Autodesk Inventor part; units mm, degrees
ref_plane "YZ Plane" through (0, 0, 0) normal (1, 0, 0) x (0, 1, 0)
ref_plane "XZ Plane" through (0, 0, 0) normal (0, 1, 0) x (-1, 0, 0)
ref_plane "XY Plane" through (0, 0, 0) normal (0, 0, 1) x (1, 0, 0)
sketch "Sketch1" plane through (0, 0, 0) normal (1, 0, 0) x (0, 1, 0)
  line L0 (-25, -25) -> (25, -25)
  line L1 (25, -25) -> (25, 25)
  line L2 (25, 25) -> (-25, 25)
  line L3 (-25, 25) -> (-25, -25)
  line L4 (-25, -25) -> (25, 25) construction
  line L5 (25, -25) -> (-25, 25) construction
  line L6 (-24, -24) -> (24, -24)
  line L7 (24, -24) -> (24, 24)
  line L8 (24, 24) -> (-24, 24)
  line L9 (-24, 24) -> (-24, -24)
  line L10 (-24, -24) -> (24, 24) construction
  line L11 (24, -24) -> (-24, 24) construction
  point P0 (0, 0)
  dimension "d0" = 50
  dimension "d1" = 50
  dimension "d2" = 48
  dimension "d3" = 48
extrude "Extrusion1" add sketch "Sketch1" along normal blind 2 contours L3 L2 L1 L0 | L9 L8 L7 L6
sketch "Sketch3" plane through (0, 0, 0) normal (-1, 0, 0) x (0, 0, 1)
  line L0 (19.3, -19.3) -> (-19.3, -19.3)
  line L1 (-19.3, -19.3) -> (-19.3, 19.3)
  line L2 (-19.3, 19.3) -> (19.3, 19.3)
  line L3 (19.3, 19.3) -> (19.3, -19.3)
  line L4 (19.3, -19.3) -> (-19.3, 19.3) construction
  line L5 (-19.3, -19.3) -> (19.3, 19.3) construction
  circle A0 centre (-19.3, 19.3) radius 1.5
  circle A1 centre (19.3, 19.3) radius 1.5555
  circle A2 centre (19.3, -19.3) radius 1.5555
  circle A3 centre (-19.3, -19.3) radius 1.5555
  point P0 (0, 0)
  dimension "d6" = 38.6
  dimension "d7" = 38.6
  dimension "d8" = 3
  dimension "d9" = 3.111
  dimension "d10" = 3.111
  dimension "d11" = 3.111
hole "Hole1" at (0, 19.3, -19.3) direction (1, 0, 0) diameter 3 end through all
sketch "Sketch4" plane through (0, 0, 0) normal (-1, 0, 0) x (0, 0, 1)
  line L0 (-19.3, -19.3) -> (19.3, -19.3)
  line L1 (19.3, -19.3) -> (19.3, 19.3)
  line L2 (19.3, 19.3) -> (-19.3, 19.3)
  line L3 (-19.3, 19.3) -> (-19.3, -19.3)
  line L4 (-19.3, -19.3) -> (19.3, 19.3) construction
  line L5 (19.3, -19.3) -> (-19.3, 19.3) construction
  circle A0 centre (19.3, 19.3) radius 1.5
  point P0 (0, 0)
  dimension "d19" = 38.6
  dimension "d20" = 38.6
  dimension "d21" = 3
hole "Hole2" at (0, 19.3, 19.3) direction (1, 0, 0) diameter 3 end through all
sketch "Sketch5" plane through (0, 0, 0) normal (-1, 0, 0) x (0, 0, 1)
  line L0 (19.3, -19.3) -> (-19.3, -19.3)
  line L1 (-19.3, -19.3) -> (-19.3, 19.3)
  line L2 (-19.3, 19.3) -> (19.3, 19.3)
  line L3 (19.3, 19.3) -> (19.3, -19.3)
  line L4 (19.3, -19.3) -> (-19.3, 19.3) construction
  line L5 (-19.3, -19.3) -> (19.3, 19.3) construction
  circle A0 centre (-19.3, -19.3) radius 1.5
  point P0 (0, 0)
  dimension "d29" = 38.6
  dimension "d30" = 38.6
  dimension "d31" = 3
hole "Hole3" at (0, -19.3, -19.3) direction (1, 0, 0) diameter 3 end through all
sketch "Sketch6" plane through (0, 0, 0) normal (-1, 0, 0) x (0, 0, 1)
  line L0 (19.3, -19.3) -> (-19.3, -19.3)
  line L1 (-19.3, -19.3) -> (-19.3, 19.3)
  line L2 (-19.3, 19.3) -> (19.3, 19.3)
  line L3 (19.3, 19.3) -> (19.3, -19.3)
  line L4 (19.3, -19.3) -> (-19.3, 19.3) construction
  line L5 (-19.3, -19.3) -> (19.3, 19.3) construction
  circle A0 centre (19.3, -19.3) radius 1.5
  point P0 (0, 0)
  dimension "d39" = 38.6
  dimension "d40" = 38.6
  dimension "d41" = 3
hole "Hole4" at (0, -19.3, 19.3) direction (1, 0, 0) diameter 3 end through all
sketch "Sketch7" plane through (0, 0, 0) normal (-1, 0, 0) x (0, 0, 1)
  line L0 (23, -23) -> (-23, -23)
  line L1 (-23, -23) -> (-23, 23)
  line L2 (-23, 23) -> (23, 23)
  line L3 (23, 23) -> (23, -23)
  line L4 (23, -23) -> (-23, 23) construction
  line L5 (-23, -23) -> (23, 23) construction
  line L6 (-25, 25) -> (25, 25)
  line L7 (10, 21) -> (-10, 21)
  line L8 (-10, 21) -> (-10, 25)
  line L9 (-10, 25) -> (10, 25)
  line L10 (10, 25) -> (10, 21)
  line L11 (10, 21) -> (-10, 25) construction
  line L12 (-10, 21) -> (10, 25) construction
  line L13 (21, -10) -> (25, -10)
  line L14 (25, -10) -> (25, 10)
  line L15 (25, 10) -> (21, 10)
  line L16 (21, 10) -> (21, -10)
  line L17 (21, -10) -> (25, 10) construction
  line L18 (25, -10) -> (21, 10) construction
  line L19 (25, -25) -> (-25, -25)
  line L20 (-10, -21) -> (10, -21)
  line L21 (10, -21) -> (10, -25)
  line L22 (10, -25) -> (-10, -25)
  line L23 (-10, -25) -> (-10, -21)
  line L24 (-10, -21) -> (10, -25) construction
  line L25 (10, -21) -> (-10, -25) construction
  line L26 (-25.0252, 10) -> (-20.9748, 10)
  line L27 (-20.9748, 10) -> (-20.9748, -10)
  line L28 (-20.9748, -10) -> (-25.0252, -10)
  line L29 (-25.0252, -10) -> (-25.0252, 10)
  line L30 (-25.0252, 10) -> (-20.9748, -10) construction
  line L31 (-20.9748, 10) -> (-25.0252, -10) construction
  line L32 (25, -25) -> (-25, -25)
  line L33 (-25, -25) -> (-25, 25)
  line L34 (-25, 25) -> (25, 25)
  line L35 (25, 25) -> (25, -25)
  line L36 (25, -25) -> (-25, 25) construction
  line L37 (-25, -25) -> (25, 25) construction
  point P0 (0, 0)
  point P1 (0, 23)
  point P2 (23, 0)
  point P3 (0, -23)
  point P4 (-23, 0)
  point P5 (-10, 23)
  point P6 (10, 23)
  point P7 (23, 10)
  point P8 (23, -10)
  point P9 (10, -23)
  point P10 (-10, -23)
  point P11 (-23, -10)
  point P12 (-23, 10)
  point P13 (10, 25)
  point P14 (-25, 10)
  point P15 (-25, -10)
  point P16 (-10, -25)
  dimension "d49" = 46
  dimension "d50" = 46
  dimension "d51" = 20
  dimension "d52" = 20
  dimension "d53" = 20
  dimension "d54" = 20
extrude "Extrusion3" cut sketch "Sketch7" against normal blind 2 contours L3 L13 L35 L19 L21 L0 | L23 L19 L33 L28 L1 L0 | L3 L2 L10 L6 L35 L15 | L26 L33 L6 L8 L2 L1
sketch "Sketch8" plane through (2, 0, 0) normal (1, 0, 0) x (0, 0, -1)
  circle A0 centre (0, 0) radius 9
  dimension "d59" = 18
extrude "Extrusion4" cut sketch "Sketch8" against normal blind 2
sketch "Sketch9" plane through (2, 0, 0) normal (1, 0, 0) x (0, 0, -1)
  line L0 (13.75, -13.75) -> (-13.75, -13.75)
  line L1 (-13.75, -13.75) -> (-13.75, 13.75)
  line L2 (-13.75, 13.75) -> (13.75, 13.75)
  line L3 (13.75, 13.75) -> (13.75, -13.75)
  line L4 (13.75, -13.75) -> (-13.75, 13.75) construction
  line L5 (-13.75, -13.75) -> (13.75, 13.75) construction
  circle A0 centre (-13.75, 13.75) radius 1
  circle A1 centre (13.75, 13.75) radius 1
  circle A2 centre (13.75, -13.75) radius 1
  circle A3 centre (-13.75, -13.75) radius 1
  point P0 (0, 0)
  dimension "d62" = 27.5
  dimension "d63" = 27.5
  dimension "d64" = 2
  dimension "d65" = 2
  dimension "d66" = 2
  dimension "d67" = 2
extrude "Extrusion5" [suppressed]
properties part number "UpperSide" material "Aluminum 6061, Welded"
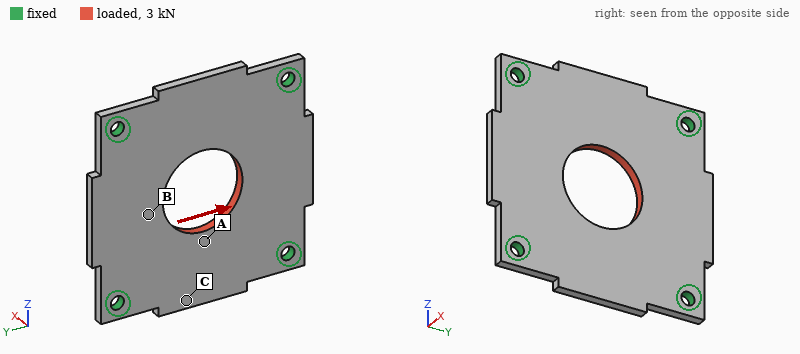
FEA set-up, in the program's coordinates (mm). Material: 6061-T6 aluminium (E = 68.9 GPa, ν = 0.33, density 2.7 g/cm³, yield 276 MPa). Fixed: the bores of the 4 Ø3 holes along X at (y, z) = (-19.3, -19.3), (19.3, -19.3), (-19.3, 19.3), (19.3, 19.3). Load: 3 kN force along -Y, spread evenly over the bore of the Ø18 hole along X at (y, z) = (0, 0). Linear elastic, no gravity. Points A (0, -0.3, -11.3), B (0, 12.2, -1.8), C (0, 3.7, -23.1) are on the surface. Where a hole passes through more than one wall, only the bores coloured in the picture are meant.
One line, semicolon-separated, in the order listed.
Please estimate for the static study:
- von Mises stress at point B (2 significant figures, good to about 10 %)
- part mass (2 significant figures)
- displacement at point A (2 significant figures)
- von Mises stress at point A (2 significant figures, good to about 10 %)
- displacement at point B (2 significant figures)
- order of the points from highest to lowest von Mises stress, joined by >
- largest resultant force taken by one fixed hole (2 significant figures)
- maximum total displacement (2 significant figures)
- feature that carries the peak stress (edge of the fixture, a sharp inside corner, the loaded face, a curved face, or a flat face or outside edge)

21 MPa; 11 g; 9.6 µm; 41 MPa; 14 µm; A > B > C; 810 N; 15 µm; edge of the fixture
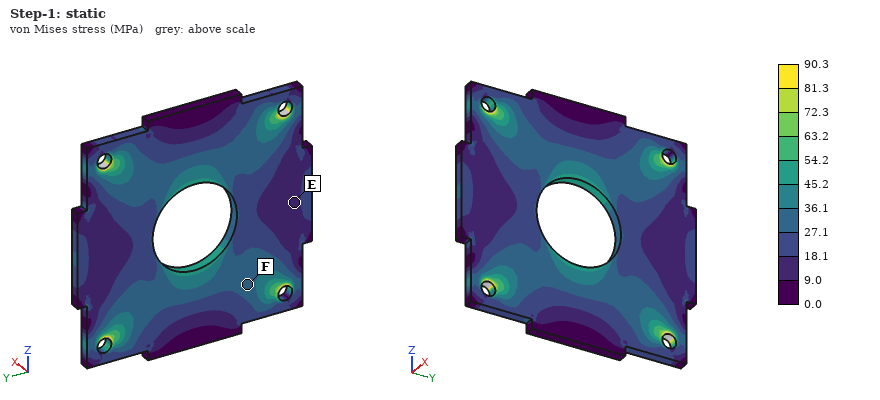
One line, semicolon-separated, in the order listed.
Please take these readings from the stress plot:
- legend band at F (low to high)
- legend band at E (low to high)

27.1 to 36.1 MPa; 9.0 to 18.1 MPa
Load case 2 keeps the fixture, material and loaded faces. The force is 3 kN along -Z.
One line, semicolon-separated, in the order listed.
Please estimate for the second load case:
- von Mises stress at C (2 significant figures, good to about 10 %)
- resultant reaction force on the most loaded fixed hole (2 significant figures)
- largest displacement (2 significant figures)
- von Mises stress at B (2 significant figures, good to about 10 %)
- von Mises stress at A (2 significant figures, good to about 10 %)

18 MPa; 810 N; 15 µm; 37 MPa; 22 MPa
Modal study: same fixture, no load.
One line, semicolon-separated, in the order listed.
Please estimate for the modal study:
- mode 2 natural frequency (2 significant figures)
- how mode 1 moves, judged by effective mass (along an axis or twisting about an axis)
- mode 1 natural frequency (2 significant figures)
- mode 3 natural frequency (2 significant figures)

7300 Hz; along X; 5200 Hz; 7300 Hz
